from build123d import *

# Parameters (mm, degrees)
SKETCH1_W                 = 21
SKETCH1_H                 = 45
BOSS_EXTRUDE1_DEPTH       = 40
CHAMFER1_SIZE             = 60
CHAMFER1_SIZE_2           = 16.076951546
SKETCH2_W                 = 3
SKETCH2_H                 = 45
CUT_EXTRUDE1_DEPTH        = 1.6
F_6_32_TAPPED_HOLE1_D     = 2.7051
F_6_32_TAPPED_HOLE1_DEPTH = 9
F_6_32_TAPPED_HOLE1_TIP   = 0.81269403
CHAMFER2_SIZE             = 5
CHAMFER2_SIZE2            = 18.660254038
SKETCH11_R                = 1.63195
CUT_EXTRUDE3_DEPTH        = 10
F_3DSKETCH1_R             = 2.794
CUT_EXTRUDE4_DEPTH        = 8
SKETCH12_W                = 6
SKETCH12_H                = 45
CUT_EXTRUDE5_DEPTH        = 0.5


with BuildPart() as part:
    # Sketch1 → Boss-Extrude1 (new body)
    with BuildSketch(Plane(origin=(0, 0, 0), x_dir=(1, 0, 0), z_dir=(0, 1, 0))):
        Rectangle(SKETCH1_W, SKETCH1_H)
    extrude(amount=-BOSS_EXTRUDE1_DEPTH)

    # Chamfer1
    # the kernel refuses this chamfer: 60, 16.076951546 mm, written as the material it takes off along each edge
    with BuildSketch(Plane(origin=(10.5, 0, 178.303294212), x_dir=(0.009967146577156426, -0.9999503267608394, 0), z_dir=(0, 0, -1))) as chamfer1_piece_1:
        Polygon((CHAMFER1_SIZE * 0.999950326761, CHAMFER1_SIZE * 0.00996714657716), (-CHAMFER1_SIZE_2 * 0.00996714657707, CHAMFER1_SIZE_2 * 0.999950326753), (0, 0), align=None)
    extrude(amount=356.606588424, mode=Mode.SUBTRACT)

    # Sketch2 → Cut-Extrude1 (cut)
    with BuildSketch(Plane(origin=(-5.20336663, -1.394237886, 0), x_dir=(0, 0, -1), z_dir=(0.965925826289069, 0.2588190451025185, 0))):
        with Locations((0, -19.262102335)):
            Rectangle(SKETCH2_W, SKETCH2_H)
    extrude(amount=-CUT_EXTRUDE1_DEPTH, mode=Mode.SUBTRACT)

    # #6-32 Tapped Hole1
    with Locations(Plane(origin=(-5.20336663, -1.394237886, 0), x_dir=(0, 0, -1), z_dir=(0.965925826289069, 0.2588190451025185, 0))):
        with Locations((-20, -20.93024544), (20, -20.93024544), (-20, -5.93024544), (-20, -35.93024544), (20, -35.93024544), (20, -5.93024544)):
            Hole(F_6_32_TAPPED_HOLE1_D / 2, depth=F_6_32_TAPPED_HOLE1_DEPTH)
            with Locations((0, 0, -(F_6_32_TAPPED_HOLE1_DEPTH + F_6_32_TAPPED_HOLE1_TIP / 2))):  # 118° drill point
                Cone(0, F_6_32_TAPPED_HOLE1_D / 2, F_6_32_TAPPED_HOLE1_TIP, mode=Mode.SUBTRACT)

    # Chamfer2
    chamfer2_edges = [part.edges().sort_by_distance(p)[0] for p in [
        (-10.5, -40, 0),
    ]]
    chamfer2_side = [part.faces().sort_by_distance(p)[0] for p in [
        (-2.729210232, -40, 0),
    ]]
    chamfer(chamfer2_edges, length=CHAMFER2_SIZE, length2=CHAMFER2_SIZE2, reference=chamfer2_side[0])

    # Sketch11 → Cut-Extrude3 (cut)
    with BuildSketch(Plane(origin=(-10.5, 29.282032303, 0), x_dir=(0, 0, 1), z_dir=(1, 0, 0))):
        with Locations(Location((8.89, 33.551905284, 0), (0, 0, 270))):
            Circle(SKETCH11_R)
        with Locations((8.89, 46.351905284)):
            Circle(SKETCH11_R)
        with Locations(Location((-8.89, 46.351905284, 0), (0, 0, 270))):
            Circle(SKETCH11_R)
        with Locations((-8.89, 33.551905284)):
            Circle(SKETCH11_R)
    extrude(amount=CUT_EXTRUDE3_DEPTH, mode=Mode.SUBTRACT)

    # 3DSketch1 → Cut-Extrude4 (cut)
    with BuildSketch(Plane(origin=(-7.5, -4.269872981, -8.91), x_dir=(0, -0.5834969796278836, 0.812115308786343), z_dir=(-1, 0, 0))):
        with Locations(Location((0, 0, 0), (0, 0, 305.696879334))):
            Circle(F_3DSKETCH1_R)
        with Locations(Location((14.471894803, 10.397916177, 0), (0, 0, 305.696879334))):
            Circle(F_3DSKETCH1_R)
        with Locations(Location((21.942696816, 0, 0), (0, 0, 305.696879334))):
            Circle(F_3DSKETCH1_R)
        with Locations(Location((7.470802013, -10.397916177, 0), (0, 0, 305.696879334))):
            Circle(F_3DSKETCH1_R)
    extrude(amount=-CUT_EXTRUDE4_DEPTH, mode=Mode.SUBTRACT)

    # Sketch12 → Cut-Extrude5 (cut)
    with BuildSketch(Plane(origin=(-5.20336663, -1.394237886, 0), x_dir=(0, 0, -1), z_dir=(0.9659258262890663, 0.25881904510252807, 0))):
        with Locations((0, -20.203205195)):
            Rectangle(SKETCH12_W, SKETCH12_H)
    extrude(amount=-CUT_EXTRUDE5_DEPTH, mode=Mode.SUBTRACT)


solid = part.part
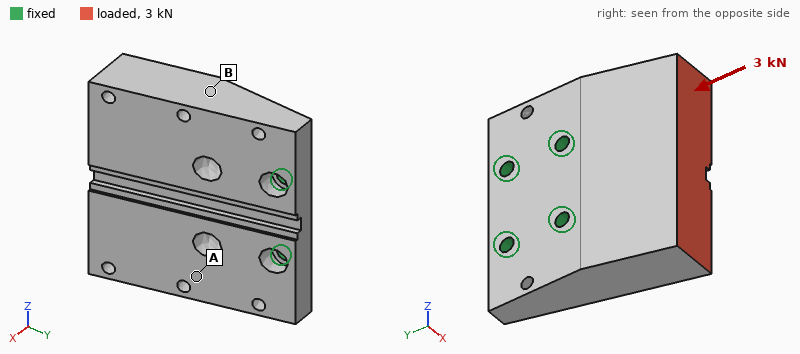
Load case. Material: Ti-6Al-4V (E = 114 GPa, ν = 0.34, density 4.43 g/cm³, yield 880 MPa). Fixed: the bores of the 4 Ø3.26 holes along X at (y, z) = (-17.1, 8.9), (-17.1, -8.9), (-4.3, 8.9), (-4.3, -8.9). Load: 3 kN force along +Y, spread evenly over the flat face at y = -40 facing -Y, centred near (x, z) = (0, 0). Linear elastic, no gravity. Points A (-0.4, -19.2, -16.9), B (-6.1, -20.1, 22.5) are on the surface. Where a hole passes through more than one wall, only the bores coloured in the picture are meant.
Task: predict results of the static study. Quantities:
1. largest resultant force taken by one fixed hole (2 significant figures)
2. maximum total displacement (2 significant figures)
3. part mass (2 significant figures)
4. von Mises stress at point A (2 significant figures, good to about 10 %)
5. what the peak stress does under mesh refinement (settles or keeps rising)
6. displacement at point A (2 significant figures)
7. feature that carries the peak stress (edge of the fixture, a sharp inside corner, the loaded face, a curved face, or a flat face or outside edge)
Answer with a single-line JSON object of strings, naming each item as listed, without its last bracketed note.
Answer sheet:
{"largest resultant force taken by one fixed hole": "1.3 kN", "maximum total displacement": "31 µm", "part mass": "68 g", "von Mises stress at point A": "35 MPa", "what the peak stress does under mesh refinement": "keeps rising", "displacement at point A": "7.9 µm", "feature that carries the peak stress": "edge of the fixture"}
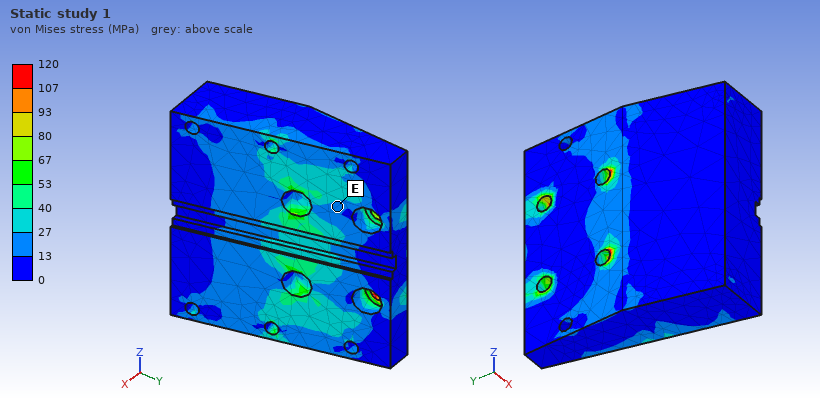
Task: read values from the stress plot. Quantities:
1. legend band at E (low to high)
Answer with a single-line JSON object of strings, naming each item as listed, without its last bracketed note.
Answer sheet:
{"legend band at E": "13 to 27 MPa"}
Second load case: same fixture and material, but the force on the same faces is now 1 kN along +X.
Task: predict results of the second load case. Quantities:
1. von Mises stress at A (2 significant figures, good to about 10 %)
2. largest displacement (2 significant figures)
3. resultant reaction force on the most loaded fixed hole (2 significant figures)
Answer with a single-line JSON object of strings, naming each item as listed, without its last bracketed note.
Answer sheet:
{"von Mises stress at A": "30 MPa", "largest displacement": "32 µm", "resultant reaction force on the most loaded fixed hole": "1.3 kN"}
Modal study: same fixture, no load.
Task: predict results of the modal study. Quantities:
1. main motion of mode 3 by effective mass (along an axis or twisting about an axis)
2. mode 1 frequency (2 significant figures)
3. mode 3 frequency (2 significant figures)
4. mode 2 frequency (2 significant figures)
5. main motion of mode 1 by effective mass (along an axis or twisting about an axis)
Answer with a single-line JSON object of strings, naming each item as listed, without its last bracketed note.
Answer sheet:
{"main motion of mode 3 by effective mass": "along Z", "mode 1 frequency": "7200 Hz", "mode 3 frequency": "14 kHz", "mode 2 frequency": "10 kHz", "main motion of mode 1 by effective mass": "along X"}
